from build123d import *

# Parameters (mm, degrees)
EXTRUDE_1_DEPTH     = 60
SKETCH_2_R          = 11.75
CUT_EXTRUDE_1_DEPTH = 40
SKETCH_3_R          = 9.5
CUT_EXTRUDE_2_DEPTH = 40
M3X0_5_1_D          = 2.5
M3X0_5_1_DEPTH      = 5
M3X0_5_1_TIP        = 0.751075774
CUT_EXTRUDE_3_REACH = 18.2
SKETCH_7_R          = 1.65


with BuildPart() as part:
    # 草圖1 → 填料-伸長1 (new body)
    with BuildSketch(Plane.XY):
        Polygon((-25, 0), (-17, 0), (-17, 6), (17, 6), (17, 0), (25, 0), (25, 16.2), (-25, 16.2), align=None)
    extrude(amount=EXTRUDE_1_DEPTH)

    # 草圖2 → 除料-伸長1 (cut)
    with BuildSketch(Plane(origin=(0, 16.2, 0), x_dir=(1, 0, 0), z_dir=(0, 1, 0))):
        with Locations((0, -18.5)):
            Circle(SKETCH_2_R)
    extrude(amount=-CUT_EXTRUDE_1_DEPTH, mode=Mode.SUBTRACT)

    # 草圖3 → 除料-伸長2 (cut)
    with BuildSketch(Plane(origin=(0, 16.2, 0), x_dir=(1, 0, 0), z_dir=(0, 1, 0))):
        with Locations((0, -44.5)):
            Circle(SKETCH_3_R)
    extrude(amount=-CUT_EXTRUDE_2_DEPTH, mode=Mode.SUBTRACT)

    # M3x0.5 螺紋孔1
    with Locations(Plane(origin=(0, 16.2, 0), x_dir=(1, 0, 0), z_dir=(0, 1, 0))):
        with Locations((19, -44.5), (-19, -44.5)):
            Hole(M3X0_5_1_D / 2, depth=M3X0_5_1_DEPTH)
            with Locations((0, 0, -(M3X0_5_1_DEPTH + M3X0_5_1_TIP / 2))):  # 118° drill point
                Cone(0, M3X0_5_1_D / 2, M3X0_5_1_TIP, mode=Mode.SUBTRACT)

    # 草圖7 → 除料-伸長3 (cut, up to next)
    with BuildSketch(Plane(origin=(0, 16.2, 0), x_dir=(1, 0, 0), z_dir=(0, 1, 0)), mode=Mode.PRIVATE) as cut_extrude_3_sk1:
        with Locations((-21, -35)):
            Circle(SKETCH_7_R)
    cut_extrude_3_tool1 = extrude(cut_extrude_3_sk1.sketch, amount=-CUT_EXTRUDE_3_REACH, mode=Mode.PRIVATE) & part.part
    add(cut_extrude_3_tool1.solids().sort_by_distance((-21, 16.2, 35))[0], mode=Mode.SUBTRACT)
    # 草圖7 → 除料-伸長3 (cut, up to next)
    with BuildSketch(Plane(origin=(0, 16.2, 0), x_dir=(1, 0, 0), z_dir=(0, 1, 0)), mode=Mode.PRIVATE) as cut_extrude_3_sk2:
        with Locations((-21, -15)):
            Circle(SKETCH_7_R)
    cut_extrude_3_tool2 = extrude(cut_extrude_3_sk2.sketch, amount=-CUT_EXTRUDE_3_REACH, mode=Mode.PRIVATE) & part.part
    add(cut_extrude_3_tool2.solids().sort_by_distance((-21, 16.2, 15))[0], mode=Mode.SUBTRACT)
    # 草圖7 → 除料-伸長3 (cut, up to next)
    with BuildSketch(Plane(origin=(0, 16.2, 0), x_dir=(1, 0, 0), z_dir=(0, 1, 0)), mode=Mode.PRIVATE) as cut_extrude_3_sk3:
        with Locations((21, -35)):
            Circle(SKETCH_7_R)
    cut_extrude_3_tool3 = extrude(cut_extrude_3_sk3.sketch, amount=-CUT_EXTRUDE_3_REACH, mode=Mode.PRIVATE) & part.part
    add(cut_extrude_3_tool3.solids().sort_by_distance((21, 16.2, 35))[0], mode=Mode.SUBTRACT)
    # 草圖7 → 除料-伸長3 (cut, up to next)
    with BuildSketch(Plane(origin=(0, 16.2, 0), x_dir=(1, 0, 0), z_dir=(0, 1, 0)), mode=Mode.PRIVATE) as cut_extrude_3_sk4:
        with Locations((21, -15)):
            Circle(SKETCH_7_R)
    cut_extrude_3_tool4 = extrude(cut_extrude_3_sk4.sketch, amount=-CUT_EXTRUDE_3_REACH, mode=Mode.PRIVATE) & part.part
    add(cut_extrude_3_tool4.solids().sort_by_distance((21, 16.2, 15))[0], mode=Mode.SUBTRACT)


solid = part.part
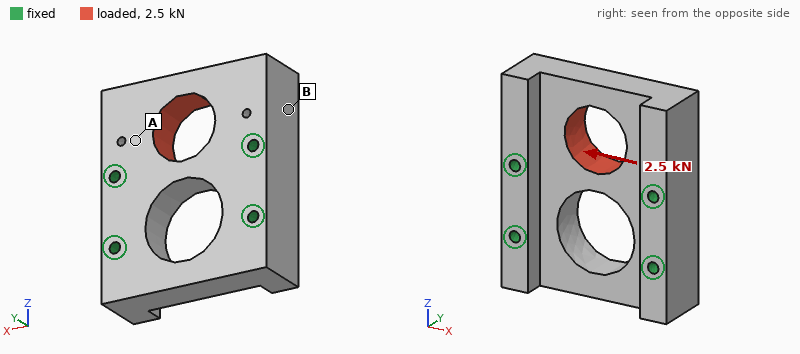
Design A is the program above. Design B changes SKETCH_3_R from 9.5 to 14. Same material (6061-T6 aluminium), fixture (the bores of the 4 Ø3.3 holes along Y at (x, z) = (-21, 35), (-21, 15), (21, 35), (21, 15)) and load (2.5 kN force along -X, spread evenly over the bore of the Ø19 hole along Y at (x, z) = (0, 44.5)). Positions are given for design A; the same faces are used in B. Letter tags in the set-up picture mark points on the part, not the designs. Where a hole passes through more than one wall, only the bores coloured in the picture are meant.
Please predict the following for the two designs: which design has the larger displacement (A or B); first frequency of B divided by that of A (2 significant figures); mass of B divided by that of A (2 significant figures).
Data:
B
0.86
0.88
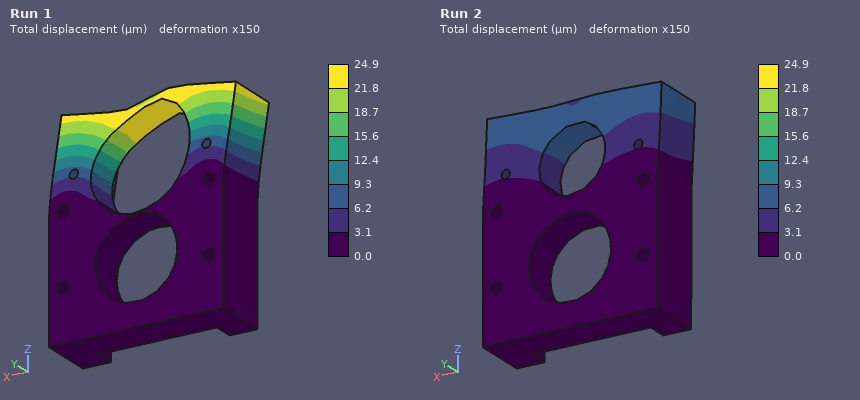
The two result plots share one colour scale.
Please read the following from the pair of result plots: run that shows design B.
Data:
Run 1
